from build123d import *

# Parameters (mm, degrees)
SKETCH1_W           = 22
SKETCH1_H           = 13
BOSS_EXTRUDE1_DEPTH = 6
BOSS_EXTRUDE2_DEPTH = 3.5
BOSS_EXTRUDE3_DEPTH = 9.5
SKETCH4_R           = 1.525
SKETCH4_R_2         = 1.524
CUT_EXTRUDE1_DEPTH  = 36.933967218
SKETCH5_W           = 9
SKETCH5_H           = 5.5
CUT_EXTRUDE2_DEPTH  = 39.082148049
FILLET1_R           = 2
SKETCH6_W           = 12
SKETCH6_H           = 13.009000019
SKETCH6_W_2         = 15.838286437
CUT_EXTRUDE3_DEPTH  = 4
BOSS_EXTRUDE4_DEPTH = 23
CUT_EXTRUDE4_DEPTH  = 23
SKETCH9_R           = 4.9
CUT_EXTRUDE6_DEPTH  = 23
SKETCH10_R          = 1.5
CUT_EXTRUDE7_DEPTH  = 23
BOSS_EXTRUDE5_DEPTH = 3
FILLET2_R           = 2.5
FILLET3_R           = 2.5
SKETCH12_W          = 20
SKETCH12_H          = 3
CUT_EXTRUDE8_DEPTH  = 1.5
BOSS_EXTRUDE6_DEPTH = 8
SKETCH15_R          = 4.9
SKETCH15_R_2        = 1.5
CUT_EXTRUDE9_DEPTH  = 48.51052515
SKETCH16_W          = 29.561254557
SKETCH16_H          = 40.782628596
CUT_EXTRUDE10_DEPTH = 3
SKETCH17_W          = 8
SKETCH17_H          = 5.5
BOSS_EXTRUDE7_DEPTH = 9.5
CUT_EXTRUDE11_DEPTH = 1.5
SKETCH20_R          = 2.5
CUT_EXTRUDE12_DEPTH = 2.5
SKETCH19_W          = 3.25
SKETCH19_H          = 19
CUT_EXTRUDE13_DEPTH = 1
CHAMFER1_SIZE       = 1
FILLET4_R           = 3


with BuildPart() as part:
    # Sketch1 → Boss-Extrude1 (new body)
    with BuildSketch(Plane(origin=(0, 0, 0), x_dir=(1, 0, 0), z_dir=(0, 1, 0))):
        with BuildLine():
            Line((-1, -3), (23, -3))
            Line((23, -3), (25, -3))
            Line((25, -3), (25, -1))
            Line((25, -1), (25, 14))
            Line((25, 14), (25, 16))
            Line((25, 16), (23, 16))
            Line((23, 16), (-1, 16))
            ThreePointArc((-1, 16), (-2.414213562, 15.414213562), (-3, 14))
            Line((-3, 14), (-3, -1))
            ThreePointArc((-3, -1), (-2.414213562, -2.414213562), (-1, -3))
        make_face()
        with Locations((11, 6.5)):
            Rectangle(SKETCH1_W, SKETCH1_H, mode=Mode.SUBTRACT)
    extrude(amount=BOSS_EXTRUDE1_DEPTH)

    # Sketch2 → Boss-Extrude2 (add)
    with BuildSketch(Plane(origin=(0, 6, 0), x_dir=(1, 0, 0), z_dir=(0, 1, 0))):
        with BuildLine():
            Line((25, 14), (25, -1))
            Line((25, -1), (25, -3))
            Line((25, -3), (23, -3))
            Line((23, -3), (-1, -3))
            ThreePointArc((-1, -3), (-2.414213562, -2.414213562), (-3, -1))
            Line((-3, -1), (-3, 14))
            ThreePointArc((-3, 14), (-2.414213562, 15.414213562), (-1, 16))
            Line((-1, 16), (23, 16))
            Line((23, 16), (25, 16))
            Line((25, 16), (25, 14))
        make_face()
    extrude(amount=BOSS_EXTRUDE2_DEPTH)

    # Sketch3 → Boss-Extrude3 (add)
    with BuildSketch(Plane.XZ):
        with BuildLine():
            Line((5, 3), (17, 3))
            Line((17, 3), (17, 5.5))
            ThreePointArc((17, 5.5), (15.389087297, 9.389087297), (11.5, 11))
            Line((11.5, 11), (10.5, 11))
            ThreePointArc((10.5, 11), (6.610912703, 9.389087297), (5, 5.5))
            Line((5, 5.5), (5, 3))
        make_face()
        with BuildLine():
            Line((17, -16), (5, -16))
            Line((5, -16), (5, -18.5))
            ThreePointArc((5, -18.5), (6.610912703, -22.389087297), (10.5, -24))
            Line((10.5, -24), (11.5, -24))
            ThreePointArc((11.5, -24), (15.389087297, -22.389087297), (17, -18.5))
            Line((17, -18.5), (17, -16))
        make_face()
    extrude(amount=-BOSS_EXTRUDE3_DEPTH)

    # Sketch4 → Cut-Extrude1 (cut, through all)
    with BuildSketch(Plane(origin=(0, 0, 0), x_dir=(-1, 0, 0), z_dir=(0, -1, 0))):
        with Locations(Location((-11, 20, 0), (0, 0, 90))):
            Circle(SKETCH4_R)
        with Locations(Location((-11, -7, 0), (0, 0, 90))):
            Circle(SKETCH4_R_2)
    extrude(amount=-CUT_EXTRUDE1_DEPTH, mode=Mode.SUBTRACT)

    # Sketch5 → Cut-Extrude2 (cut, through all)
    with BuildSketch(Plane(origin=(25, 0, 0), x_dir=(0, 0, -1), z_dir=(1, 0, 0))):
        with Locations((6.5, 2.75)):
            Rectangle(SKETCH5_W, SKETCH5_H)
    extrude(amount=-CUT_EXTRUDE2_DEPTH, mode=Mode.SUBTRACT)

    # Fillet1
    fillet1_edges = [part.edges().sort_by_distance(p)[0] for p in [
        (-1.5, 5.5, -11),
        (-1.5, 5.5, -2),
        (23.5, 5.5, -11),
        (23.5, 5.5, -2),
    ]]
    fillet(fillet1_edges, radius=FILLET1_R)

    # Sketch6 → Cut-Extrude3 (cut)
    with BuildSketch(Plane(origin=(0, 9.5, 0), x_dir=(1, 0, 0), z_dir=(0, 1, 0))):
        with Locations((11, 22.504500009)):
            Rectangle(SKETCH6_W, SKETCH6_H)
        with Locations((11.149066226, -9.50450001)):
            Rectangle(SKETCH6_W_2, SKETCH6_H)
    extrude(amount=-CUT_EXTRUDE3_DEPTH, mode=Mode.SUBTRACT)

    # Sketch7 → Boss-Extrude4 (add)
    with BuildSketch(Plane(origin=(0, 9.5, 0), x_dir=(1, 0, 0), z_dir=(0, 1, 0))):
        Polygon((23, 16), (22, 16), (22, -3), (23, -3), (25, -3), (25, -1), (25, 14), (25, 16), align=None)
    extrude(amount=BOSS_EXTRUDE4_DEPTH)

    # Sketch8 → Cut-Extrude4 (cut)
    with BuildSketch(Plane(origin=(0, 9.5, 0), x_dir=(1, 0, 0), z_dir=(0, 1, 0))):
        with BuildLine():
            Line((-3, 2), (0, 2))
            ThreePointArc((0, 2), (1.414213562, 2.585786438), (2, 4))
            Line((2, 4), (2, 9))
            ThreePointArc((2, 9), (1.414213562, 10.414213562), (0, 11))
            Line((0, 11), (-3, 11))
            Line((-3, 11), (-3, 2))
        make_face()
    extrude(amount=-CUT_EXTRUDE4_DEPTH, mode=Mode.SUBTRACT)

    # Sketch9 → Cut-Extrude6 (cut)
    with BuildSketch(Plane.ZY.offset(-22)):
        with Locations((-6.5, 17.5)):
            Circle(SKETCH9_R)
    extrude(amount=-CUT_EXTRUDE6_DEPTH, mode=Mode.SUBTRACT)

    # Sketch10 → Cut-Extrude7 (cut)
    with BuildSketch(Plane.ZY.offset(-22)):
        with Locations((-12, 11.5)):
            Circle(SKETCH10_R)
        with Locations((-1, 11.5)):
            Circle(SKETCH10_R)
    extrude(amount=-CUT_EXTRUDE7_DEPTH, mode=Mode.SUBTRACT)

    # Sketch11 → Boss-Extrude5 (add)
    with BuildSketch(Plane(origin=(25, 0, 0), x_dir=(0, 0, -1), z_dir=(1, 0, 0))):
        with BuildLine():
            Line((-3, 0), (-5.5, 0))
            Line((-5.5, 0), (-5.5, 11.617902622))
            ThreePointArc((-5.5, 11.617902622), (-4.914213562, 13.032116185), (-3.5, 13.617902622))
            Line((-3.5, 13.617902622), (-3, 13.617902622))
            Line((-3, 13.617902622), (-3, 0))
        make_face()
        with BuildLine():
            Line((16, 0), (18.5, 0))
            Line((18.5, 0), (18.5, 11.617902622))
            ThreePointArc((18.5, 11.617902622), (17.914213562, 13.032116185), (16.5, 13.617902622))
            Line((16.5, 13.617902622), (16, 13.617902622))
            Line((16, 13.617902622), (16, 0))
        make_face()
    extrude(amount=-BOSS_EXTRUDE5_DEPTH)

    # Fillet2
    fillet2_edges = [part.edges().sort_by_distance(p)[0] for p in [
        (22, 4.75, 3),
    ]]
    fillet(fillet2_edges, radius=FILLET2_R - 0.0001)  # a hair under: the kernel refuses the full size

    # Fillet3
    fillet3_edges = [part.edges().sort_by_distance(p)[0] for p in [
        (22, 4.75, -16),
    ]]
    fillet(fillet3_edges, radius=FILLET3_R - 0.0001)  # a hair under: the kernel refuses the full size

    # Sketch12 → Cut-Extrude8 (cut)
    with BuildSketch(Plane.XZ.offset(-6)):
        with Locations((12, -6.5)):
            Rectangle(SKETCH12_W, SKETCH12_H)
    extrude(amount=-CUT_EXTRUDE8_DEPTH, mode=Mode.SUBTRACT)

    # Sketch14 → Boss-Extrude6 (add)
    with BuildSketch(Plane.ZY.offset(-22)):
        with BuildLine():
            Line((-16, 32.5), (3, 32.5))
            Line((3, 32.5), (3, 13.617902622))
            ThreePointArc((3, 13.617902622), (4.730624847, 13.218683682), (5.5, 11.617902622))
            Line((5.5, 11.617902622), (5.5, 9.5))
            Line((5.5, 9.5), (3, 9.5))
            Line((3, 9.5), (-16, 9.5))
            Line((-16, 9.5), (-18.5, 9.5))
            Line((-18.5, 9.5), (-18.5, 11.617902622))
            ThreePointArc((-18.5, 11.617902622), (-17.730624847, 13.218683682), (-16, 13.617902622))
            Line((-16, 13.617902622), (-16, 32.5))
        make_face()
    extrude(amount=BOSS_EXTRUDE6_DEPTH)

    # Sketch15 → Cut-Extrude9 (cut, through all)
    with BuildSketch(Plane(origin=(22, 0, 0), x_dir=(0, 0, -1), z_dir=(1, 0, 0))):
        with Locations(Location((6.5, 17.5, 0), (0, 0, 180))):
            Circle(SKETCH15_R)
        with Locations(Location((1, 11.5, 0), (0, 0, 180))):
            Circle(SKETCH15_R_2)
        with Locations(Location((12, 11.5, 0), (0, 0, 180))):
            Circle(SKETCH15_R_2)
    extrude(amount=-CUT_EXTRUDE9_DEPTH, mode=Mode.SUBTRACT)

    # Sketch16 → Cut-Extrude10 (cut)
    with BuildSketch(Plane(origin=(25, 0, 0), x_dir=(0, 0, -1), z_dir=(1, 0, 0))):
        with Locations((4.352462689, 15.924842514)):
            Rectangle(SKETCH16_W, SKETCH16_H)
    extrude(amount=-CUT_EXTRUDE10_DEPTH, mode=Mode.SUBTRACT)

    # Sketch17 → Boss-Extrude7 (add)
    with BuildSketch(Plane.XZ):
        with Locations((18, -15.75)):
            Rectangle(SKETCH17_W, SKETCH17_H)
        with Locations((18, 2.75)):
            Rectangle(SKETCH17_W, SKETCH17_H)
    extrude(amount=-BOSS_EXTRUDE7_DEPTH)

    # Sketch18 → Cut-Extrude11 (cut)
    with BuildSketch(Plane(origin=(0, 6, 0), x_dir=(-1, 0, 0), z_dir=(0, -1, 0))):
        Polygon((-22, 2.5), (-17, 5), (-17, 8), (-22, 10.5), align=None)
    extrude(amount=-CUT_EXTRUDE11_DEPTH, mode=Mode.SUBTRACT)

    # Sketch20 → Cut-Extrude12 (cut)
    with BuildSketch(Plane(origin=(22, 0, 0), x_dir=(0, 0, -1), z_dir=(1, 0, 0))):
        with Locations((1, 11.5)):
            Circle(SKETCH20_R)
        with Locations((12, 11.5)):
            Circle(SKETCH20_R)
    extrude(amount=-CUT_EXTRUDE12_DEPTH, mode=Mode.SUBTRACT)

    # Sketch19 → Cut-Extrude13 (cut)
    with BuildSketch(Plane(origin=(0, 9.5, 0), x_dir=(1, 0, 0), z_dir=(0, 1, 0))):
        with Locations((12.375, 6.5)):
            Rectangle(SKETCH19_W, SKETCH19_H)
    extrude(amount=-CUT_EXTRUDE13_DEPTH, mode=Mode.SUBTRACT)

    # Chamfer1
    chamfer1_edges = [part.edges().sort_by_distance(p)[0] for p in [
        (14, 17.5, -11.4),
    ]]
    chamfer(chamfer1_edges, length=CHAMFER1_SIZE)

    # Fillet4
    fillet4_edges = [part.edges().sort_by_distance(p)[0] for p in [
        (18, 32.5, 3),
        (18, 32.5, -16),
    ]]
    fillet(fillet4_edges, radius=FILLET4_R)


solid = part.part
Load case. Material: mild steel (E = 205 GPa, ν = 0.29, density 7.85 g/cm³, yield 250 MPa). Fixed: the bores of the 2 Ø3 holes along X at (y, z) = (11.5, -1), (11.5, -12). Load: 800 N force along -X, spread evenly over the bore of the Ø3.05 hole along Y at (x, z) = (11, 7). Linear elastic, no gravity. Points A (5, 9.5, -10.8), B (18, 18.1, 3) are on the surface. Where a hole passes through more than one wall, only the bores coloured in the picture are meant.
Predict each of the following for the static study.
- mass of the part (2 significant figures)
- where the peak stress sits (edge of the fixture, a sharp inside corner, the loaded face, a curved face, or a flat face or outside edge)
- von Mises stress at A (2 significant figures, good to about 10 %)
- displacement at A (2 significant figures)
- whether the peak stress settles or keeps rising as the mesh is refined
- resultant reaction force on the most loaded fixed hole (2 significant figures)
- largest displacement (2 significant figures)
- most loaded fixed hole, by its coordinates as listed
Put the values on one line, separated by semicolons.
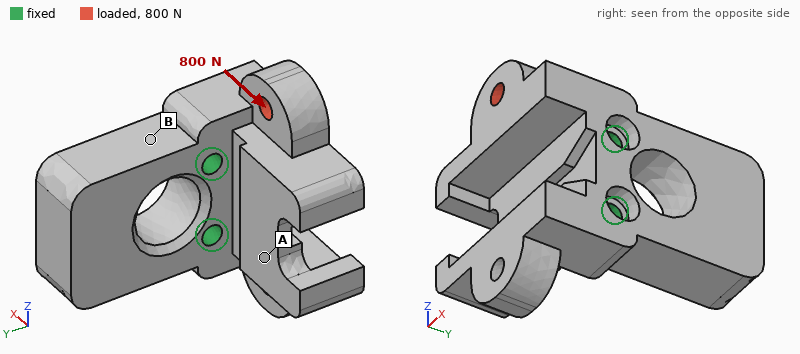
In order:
49 g; edge of the fixture; 27 MPa; 5.4 µm; keeps rising; 1.1 kN; 17 µm; (11.5, -1)
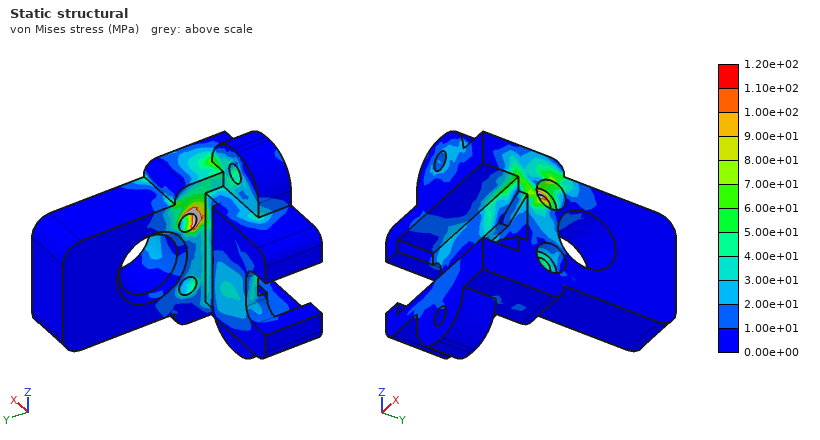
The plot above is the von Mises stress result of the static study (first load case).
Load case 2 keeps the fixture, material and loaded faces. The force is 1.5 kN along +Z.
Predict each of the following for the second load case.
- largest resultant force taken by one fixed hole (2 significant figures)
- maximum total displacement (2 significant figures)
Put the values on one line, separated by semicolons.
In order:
1.2 kN; 28 µm
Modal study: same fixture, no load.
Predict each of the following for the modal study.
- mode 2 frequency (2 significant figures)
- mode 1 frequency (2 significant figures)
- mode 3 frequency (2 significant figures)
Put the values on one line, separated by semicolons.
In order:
10000 Hz; 8200 Hz; 11 kHz
